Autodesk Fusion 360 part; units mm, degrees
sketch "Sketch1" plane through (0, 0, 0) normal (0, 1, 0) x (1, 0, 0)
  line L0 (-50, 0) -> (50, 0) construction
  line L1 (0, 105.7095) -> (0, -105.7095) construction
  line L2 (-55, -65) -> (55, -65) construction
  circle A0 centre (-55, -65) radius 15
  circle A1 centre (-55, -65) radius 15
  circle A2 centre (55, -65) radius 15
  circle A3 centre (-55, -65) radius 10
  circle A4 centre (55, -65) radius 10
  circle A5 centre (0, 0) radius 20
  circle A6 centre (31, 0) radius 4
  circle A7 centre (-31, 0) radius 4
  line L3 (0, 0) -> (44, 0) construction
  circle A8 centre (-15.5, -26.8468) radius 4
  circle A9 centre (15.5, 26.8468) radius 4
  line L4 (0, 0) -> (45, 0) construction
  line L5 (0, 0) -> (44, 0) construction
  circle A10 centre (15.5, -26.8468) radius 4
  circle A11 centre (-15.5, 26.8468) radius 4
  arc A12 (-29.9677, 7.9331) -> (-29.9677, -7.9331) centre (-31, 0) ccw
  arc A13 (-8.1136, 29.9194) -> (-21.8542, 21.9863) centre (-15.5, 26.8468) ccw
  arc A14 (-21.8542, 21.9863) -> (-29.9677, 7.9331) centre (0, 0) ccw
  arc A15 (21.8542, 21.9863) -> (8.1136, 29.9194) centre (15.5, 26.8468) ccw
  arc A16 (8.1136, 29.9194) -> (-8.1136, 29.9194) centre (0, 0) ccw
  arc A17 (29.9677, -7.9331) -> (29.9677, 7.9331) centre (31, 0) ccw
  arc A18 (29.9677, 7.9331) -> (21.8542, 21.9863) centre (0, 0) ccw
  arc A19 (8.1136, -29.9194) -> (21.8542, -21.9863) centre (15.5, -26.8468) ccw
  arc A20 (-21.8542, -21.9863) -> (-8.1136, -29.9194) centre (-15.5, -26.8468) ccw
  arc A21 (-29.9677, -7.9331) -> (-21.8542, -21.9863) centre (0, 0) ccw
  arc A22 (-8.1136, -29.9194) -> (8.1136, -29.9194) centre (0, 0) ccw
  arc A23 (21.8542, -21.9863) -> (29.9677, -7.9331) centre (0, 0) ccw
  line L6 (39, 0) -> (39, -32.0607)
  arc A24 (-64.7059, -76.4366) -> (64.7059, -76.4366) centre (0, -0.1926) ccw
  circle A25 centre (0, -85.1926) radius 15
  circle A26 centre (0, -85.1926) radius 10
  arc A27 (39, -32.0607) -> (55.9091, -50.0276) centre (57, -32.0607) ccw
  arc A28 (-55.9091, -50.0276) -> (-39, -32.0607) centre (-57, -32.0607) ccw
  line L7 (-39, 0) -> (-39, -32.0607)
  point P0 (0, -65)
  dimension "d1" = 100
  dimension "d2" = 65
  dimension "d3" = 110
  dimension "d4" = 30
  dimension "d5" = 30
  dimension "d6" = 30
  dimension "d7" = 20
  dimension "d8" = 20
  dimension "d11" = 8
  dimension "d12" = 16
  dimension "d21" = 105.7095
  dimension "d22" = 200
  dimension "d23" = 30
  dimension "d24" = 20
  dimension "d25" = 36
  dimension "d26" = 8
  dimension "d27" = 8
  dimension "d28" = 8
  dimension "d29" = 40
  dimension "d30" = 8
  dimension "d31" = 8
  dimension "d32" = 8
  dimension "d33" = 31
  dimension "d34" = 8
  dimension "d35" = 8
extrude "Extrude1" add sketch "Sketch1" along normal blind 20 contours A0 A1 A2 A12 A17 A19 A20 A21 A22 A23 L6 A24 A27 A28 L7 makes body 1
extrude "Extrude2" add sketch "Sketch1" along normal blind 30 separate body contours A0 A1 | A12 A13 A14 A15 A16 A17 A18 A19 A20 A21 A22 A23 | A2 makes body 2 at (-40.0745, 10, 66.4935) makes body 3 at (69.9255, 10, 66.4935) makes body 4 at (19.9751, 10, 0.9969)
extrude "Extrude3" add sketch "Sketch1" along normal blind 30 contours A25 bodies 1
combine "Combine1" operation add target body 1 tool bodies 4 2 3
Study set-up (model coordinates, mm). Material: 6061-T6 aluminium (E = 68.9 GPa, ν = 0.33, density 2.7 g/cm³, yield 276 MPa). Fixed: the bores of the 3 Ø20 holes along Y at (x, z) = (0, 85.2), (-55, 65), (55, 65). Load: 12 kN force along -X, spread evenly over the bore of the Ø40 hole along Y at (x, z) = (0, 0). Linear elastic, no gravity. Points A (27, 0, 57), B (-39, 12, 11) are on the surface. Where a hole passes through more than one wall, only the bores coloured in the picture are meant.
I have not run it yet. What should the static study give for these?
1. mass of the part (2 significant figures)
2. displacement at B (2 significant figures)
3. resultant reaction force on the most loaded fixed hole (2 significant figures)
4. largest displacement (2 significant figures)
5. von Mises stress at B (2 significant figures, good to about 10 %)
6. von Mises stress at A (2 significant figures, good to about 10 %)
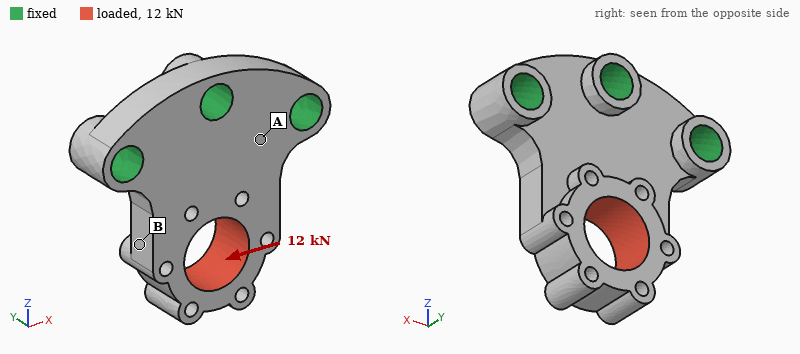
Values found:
580 g
38 µm
9.4 kN
84 µm
25 MPa
7.1 MPa
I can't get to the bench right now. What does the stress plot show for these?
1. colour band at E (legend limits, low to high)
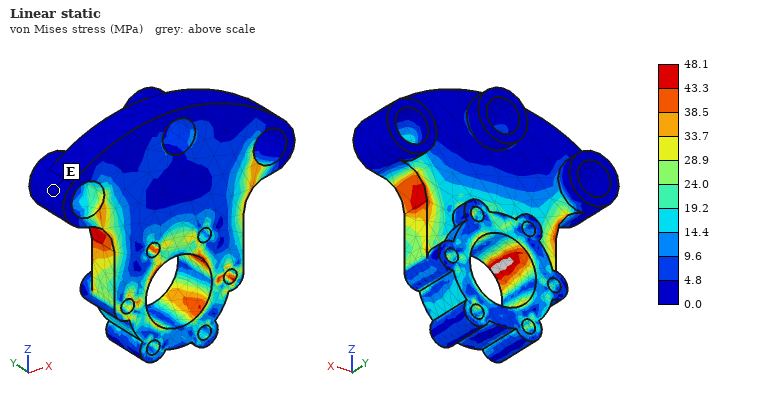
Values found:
0.0 to 4.8 MPa
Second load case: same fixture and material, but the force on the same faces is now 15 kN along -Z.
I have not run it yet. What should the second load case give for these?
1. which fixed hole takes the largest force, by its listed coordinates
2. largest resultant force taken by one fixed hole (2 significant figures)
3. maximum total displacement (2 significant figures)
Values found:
(0, 85.2)
7.4 kN
89 µm
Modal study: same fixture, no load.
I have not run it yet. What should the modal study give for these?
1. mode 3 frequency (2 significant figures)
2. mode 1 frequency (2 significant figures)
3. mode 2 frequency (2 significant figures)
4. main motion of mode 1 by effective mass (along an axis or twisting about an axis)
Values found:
5200 Hz
1900 Hz
5100 Hz
along Y
